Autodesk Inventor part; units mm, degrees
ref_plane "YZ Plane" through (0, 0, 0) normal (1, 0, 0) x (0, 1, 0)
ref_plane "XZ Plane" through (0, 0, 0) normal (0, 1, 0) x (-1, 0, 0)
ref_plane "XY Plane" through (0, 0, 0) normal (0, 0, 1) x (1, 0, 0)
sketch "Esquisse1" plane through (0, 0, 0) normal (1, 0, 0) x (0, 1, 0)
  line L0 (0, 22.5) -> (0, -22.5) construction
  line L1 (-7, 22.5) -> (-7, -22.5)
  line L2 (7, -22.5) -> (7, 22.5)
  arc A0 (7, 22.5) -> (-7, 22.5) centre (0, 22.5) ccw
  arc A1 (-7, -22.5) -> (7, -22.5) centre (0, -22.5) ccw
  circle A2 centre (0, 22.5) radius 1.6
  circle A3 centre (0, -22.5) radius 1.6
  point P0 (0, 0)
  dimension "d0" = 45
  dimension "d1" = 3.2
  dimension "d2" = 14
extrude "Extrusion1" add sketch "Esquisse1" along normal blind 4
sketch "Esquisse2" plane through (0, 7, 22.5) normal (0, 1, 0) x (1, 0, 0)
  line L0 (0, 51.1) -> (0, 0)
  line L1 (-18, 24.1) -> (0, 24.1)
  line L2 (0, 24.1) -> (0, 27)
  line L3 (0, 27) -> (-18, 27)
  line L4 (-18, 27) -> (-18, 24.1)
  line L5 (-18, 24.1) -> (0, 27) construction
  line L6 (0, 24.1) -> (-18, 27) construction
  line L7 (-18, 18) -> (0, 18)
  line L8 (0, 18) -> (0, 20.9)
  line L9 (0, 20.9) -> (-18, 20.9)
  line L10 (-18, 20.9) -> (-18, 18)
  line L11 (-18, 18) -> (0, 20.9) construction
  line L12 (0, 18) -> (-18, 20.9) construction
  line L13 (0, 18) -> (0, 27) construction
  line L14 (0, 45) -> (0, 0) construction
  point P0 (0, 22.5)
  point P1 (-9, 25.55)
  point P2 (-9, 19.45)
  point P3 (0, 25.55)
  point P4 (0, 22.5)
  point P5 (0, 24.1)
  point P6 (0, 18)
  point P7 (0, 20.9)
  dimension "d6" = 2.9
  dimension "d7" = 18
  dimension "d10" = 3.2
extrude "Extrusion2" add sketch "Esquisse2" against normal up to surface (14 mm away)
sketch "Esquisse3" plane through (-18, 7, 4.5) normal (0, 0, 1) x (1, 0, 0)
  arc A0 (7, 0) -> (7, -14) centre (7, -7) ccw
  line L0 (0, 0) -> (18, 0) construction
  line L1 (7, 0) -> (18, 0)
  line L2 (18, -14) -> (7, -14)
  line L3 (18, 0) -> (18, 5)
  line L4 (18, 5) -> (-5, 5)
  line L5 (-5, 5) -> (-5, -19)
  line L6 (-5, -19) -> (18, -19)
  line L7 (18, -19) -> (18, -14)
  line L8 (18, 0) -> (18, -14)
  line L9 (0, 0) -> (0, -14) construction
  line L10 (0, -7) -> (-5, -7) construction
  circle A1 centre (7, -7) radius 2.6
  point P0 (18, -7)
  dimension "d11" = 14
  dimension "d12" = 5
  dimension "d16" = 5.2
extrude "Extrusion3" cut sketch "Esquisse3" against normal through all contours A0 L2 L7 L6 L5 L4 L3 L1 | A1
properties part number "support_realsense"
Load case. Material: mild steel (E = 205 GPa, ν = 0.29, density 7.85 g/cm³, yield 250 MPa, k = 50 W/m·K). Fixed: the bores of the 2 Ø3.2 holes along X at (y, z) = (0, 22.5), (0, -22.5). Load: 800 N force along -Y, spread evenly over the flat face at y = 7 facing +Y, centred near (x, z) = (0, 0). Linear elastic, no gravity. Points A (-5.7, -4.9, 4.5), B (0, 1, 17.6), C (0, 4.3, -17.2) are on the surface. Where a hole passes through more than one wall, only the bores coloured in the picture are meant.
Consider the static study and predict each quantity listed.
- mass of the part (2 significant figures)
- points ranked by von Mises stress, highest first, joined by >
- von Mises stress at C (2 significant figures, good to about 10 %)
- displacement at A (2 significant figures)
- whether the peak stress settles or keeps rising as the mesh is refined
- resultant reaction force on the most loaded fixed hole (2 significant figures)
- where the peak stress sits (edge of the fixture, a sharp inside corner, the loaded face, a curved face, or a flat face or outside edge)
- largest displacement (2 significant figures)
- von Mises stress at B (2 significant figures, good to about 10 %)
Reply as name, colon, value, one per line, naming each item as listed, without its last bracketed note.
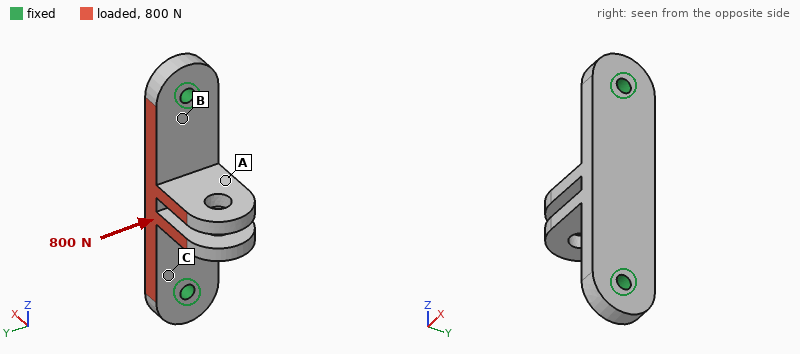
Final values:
mass of the part: 34 g
points ranked by von Mises stress, highest first, joined by >: B > C > A
von Mises stress at C: 26 MPa
displacement at A: 10 µm
whether the peak stress settles or keeps rising as the mesh is refined: keeps rising
resultant reaction force on the most loaded fixed hole: 400 N
where the peak stress sits: edge of the fixture
largest displacement: 19 µm
von Mises stress at B: 35 MPa
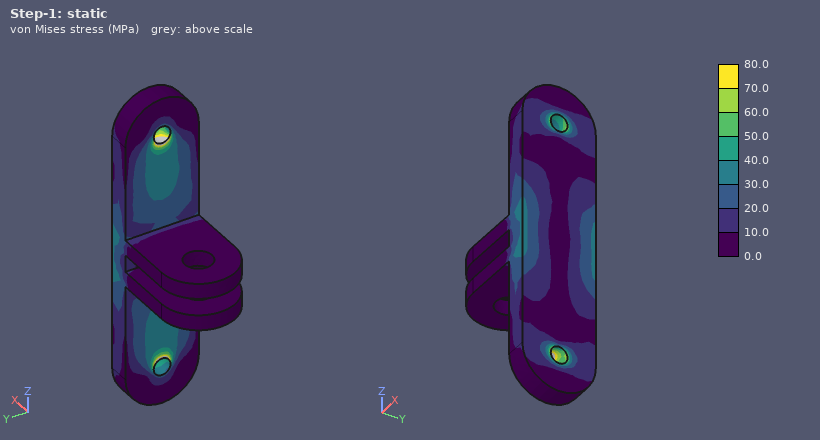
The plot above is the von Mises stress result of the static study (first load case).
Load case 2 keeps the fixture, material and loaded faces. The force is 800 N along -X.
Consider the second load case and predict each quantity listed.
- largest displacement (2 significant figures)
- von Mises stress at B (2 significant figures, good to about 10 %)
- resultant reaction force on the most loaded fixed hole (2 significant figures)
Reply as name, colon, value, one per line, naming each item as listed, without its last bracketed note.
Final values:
largest displacement: 41 µm
von Mises stress at B: 73 MPa
resultant reaction force on the most loaded fixed hole: 400 N
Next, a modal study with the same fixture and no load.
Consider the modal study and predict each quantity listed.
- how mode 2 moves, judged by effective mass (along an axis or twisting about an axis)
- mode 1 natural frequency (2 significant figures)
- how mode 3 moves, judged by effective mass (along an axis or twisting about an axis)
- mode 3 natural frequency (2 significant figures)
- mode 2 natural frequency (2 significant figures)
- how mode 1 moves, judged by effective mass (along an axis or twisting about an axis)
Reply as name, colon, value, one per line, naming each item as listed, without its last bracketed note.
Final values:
how mode 2 moves, judged by effective mass: along X
mode 1 natural frequency: 5800 Hz
how mode 3 moves, judged by effective mass: along Z
mode 3 natural frequency: 7100 Hz
mode 2 natural frequency: 6500 Hz
how mode 1 moves, judged by effective mass: along Y
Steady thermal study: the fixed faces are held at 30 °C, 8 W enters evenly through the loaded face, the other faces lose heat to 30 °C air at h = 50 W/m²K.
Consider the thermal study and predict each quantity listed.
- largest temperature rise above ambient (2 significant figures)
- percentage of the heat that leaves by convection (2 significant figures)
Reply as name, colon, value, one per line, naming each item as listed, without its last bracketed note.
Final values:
largest temperature rise above ambient: 19 K
percentage of the heat that leaves by convection: 20 %
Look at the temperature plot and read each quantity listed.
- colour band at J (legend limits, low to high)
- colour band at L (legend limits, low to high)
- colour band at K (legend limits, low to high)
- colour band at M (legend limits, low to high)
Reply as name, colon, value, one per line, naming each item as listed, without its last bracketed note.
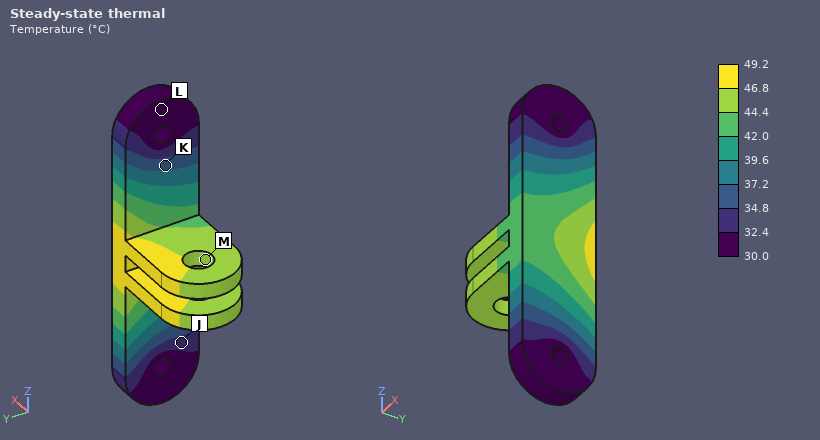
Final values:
colour band at J: 32.4 to 34.8 °C
colour band at L: 30.0 to 32.4 °C
colour band at K: 34.8 to 37.2 °C
colour band at M: 44.4 to 46.8 °C
